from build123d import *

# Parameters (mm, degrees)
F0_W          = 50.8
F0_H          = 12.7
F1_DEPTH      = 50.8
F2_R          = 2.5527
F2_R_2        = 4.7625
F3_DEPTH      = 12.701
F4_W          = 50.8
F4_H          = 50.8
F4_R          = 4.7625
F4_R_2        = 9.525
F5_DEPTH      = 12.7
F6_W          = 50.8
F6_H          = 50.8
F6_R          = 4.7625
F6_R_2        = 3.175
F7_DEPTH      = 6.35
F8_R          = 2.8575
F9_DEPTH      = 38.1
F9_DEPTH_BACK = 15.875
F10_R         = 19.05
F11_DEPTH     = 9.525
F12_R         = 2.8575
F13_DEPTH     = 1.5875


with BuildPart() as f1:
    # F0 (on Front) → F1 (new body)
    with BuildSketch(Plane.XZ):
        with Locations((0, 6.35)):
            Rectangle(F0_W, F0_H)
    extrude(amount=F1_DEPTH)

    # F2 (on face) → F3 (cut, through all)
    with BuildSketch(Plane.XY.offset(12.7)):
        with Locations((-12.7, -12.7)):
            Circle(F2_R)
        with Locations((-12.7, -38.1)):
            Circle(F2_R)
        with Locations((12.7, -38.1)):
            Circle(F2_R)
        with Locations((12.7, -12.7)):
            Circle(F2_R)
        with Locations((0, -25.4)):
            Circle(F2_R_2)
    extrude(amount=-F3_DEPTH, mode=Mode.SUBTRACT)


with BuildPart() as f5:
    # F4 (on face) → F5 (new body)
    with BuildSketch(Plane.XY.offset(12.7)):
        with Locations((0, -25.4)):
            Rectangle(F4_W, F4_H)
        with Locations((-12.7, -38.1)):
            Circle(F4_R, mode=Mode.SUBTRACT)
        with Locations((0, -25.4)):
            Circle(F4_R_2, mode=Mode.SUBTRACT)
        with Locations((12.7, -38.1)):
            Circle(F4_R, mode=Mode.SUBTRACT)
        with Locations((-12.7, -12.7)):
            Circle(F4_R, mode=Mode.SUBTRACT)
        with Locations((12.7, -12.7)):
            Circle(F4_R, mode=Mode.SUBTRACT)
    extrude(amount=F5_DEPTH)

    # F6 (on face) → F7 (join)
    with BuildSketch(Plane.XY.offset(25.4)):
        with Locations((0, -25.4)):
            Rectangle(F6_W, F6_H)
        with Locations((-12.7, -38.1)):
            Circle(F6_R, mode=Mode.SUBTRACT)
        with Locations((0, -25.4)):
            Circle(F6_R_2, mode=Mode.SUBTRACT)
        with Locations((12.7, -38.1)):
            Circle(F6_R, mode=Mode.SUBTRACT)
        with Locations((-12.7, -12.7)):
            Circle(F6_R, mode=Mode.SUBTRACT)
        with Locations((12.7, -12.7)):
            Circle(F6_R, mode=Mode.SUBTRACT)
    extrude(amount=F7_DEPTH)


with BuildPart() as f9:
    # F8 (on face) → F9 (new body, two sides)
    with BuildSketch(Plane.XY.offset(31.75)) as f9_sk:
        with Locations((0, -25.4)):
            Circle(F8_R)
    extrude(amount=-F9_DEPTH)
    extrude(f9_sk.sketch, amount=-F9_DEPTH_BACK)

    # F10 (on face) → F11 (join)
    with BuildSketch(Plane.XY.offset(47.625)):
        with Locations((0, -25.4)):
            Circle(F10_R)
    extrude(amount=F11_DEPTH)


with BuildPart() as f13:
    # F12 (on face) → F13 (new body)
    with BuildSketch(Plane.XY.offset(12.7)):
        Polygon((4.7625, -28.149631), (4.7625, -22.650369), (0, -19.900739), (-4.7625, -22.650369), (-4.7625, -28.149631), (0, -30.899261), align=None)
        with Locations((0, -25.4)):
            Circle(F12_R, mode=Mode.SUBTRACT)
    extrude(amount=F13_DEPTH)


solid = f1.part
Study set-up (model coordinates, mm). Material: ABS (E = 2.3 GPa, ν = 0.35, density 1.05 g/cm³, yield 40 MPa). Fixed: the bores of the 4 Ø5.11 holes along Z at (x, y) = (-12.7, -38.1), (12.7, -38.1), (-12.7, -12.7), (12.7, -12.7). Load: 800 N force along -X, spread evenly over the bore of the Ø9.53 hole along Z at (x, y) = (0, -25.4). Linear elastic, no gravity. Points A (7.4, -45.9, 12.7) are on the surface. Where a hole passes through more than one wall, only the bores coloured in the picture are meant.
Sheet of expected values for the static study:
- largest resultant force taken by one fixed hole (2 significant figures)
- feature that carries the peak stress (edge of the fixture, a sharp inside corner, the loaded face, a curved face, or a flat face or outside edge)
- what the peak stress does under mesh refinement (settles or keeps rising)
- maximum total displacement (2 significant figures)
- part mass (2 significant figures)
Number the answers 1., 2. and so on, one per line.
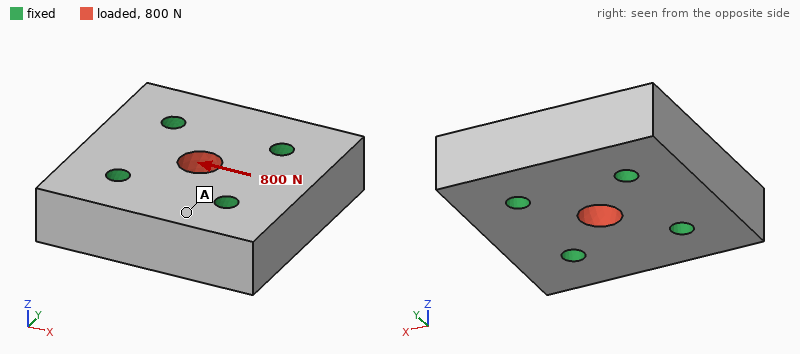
1. 210 N
2. edge of the fixture
3. keeps rising
4. 13 µm
5. 32 g
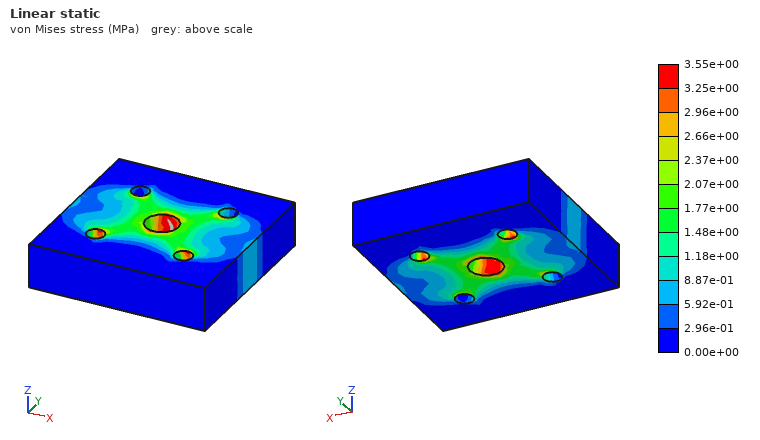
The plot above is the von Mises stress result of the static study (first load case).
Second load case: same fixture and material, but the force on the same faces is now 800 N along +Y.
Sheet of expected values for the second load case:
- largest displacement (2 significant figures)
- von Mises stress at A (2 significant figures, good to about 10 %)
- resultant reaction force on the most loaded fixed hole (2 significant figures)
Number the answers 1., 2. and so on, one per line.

1. 12 µm
2. 0.68 MPa
3. 210 N
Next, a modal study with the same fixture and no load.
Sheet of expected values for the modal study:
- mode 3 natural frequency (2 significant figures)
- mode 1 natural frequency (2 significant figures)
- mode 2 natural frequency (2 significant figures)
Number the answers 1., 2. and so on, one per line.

1. 10 kHz
2. 10 kHz
3. 10 kHz
